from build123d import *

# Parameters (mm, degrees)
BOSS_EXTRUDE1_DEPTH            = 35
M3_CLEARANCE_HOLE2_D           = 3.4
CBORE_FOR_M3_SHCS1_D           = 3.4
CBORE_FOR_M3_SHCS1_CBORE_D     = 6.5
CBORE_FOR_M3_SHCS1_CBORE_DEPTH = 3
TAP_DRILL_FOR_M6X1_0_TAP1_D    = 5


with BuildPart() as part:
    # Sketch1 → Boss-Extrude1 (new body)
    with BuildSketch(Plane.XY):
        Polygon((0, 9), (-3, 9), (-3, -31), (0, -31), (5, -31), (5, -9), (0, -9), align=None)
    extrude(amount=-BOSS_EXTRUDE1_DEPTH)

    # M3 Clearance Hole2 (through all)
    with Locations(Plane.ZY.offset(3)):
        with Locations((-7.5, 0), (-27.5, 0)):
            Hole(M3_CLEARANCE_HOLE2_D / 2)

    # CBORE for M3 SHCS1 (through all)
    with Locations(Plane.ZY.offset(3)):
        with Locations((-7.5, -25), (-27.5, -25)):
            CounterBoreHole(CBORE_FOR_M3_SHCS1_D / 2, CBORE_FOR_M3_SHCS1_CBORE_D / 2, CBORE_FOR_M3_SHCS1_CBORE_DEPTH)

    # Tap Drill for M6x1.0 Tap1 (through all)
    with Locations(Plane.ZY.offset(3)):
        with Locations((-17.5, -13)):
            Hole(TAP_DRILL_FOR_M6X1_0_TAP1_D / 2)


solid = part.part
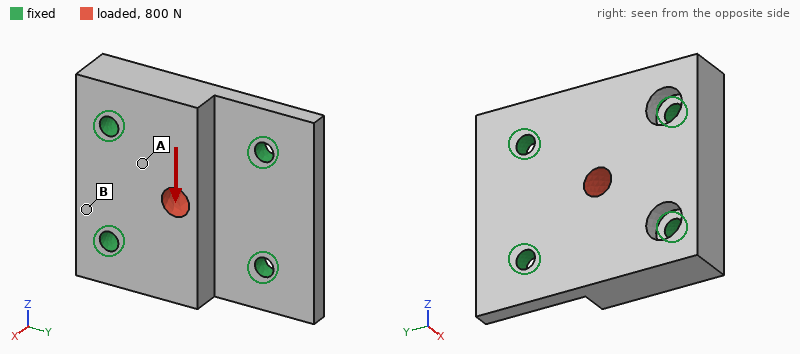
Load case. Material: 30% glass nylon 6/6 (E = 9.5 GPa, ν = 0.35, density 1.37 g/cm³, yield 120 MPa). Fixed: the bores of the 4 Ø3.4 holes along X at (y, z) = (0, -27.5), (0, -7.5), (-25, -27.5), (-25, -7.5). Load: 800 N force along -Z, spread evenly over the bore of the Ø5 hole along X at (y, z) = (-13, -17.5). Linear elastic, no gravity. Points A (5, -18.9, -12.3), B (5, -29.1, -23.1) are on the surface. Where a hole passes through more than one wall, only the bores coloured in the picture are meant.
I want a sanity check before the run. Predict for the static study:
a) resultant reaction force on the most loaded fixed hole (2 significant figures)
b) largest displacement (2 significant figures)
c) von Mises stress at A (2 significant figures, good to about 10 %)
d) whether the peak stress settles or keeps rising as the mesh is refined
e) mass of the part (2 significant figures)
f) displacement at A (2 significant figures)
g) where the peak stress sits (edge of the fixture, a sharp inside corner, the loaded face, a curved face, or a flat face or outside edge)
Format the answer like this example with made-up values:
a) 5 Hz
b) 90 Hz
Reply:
a) 290 N
b) 15 µm
c) 5.6 MPa
d) keeps rising
e) 10 g
f) 5.6 µm
g) edge of the fixture
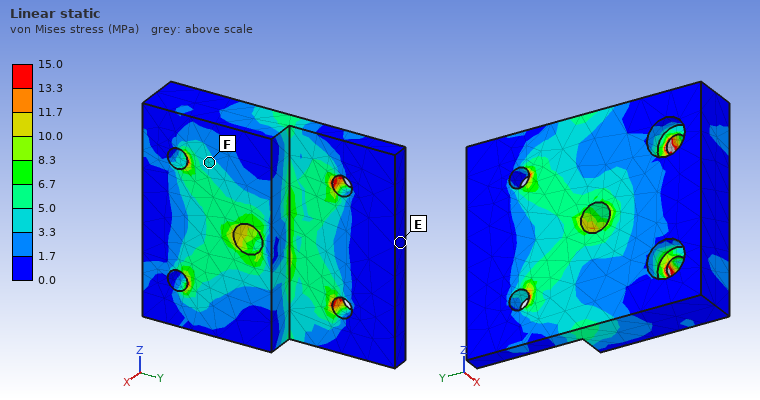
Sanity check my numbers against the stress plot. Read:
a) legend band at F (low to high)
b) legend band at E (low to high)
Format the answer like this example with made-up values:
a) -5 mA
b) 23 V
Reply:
a) 3.3 to 5.0 MPa
b) 0.0 to 1.7 MPa
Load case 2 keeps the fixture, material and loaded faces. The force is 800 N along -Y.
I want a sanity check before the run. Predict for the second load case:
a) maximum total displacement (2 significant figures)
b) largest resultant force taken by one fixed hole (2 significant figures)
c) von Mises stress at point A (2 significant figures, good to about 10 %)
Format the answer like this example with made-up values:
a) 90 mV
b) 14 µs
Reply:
a) 19 µm
b) 290 N
c) 5.8 MPa
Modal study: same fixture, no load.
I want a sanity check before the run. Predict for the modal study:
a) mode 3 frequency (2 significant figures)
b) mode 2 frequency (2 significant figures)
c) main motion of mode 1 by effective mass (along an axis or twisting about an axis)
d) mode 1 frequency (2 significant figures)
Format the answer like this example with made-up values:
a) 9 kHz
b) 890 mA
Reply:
a) 14 kHz
b) 14 kHz
c) along X
d) 12 kHz
